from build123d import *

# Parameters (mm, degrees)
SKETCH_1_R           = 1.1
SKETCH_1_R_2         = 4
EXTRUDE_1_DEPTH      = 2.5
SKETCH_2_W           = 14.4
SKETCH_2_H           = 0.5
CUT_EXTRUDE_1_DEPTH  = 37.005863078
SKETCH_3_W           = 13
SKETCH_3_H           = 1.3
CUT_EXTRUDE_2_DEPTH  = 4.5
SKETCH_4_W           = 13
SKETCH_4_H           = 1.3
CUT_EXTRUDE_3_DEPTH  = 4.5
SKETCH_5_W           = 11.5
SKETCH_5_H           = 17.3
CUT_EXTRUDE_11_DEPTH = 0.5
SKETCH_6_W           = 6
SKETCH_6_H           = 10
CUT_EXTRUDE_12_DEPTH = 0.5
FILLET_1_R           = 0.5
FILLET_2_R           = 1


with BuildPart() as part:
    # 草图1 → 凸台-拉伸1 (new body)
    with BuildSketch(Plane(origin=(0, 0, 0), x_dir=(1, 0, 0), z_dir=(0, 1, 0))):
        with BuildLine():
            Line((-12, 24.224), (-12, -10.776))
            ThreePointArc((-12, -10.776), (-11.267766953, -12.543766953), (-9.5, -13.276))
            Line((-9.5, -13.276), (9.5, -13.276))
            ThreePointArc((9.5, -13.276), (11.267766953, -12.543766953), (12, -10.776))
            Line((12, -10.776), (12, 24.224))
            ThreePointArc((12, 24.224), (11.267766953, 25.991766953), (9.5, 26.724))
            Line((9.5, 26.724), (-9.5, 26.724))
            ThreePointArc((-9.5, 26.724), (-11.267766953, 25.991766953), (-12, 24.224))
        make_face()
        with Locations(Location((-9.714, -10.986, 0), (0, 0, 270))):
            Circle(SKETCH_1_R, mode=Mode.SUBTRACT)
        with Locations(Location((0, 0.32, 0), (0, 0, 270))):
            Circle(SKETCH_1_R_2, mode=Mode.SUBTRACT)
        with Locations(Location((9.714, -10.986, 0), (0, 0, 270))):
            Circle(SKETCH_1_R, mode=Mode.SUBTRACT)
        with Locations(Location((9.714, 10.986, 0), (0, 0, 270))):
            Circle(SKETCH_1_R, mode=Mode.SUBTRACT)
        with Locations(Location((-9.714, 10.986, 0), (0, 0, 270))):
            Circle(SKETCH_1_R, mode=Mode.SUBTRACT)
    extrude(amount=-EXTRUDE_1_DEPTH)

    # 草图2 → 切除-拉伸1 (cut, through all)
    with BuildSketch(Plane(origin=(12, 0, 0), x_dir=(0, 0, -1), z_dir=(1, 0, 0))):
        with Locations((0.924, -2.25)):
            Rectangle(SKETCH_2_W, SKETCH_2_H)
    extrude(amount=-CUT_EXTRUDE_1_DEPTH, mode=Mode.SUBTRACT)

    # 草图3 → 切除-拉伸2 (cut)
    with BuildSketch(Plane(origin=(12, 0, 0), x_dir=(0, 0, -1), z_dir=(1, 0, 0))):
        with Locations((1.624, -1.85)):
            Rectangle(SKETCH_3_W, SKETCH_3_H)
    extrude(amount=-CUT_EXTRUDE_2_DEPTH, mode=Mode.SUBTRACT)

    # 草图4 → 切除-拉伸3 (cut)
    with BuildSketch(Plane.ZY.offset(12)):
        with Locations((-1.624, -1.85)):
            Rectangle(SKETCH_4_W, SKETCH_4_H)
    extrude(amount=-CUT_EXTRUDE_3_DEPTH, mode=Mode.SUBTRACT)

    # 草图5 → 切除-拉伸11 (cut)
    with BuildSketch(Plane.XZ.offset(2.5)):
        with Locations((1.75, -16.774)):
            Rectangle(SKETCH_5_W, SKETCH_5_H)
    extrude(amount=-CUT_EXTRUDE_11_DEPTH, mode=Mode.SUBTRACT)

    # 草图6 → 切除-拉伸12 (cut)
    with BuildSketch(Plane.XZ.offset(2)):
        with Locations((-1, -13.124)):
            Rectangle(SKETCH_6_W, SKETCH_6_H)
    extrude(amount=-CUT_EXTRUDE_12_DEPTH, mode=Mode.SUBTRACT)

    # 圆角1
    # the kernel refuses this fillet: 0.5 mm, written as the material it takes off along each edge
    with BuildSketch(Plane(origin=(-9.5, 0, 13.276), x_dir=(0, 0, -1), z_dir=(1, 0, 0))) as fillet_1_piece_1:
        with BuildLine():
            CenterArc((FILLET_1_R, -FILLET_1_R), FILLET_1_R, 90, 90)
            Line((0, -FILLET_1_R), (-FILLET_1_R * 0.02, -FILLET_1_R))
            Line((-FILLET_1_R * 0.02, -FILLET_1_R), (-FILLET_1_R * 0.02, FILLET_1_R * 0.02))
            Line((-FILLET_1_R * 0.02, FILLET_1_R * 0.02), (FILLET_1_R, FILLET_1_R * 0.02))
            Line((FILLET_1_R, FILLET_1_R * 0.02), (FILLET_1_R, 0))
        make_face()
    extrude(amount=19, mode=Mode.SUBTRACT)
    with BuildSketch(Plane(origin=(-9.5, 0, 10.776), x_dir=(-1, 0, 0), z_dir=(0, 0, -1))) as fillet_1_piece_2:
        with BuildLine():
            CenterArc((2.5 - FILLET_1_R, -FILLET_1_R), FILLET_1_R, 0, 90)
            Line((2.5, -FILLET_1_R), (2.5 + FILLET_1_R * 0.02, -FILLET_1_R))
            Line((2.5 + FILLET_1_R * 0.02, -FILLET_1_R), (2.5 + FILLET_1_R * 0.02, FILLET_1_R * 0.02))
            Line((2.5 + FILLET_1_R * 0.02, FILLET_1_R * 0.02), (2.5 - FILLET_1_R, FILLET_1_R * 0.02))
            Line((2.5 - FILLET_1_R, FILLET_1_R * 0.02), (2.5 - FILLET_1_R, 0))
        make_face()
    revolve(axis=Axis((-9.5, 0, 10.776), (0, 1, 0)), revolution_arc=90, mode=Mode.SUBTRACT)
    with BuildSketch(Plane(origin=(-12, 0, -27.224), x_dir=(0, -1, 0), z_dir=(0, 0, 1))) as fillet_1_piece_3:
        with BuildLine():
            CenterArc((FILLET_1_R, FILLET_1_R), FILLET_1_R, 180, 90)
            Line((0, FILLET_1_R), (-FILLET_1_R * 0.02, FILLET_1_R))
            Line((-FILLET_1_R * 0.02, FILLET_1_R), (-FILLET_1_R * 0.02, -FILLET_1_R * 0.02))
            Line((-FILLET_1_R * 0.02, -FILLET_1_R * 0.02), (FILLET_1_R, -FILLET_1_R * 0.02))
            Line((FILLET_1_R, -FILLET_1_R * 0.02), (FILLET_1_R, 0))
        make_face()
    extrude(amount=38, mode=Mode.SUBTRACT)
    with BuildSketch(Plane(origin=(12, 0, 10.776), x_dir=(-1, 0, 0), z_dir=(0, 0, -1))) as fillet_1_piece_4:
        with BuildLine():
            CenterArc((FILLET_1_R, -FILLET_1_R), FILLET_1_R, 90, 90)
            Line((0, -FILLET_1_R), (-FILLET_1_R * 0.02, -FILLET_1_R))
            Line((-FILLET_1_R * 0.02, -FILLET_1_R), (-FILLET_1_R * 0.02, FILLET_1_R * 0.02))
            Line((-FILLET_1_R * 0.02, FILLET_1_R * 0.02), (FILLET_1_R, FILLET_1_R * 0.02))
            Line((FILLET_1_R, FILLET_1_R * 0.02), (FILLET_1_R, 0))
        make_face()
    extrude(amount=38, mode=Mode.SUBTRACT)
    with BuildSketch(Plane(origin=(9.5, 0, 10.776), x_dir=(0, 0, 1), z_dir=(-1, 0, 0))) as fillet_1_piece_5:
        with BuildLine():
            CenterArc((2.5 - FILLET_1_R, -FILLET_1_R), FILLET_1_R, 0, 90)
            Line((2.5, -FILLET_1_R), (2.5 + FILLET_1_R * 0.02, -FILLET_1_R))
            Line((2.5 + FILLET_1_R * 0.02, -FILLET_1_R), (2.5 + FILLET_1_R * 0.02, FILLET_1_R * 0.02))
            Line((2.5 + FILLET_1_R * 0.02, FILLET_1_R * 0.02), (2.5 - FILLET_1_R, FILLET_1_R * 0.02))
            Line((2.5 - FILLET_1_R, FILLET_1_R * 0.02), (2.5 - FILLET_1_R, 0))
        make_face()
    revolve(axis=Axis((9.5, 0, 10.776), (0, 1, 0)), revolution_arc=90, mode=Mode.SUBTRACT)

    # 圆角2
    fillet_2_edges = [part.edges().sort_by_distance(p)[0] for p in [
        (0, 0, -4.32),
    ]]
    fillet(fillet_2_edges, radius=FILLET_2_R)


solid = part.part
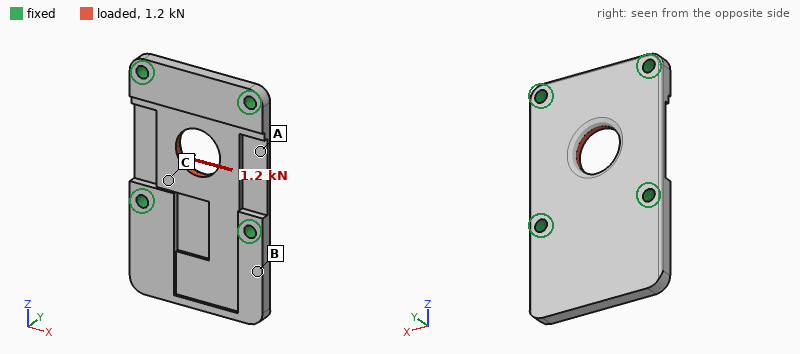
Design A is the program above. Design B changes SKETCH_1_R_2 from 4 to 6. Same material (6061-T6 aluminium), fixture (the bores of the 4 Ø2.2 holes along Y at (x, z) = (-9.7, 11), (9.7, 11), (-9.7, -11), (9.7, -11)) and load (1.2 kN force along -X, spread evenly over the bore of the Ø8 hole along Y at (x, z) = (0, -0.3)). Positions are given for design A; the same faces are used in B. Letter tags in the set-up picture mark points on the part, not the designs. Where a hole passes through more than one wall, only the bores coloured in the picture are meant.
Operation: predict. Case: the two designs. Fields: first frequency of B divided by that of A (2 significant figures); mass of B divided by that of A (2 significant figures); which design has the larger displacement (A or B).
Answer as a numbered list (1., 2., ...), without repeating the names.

1. 0.99
2. 0.93
3. B
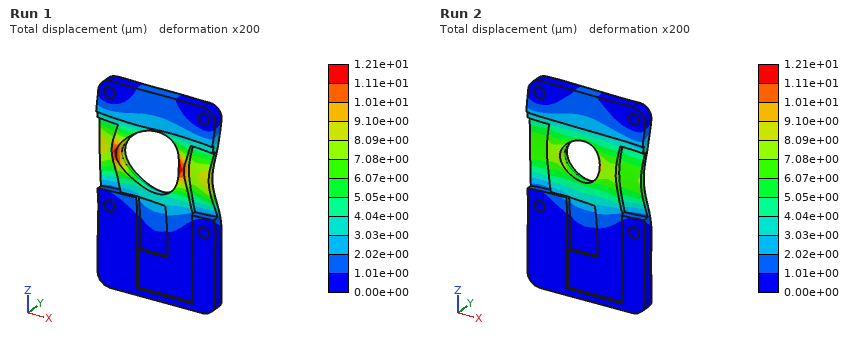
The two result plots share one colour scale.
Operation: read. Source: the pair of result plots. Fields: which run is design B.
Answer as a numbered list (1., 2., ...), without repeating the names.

1. Run 1
